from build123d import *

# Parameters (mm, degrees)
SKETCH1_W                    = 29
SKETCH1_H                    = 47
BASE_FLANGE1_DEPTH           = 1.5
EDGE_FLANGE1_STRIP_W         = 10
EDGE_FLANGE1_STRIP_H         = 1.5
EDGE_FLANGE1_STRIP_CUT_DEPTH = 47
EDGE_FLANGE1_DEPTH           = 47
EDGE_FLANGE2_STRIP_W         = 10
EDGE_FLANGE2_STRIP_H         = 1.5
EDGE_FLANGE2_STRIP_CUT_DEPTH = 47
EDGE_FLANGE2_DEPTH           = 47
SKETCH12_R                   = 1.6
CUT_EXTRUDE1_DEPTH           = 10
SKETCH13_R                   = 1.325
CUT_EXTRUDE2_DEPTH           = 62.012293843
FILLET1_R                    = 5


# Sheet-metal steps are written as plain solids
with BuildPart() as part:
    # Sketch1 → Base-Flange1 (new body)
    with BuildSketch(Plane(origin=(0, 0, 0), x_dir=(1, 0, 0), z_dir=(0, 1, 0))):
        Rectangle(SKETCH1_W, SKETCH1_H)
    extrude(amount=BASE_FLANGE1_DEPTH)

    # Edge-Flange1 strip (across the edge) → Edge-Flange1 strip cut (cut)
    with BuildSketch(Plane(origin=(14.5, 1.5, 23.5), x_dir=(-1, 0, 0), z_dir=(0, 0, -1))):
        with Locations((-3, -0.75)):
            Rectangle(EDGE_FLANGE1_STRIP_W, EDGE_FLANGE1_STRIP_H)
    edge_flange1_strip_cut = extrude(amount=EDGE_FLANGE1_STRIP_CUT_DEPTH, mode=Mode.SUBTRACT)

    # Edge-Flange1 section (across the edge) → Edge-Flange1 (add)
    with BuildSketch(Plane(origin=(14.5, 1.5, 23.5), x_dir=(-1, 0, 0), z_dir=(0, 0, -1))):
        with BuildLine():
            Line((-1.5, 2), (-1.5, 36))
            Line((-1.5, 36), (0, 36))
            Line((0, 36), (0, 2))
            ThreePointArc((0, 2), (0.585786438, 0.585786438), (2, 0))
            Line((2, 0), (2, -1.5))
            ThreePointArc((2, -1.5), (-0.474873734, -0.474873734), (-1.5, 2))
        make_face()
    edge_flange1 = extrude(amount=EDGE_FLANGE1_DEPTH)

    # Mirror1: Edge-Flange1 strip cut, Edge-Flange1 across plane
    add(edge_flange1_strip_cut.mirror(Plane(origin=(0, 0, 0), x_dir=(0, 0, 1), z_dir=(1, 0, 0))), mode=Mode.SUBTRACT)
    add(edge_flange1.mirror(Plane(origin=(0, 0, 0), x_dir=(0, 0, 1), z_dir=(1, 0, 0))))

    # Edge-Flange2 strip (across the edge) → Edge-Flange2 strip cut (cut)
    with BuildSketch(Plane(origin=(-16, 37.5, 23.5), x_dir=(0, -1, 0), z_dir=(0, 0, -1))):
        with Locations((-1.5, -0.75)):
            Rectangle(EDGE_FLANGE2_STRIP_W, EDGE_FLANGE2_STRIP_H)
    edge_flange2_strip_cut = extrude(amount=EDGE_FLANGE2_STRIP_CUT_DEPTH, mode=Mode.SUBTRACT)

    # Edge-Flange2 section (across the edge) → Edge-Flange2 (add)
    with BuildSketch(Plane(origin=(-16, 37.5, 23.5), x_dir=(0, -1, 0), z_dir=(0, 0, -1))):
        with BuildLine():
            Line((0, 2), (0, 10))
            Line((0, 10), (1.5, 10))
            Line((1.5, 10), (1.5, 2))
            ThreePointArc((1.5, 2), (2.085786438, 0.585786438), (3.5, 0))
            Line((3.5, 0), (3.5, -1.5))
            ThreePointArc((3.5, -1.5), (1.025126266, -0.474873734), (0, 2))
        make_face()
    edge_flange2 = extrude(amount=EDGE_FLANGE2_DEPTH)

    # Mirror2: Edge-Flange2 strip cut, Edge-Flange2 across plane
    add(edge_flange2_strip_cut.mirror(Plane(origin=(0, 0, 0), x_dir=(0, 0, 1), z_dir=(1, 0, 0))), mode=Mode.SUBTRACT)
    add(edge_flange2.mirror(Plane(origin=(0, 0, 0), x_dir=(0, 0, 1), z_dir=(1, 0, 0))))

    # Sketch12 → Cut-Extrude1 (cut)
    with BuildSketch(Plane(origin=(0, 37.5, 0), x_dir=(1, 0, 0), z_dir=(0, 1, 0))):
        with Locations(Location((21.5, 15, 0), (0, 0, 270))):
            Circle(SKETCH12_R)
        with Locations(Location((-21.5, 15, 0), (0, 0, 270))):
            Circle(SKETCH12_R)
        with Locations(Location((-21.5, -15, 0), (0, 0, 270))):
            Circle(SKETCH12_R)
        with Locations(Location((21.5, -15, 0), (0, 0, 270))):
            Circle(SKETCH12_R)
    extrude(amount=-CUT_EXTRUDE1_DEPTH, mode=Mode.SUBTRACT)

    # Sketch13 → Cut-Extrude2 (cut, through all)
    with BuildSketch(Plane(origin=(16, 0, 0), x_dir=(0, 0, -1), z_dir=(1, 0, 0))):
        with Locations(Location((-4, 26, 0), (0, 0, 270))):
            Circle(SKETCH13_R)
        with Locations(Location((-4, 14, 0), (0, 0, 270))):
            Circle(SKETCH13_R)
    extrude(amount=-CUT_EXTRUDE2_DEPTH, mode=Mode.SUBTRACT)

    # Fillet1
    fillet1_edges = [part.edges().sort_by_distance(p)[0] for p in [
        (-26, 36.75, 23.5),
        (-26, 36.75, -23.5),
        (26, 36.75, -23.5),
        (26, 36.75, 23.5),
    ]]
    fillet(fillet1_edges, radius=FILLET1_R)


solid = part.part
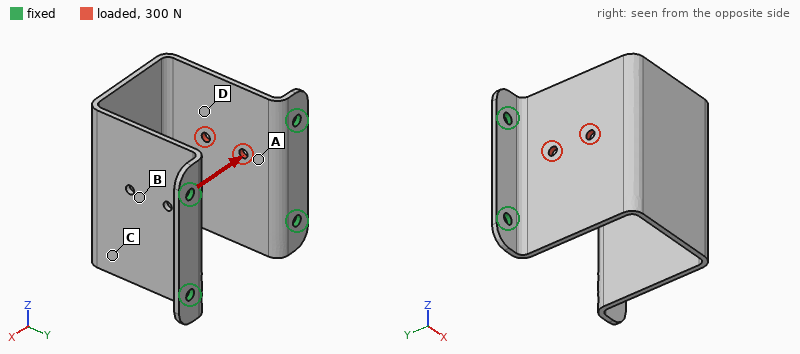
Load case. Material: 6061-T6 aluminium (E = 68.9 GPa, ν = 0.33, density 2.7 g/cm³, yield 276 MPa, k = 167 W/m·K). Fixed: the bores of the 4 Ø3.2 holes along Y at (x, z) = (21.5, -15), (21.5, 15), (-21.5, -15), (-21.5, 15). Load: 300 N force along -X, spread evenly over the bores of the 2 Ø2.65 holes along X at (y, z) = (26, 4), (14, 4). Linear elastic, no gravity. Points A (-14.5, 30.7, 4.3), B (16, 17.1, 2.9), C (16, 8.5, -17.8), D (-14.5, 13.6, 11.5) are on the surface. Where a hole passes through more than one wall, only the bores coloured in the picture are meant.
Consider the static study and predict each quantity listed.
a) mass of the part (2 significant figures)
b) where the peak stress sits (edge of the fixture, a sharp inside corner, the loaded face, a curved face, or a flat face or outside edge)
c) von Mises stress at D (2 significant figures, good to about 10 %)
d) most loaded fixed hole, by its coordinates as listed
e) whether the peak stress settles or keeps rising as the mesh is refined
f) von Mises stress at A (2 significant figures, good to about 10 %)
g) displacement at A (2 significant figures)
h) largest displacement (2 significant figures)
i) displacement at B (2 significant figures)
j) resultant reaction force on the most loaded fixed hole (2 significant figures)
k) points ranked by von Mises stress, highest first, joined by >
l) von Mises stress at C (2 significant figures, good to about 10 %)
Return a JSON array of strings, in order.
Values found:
["22 g", "edge of the fixture", "85 MPa", "(-21.5, 15)", "keeps rising", "59 MPa", "0.15 mm", "0.49 mm", "0.26 mm", "150 N", "D > A > C > B", "33 MPa"]
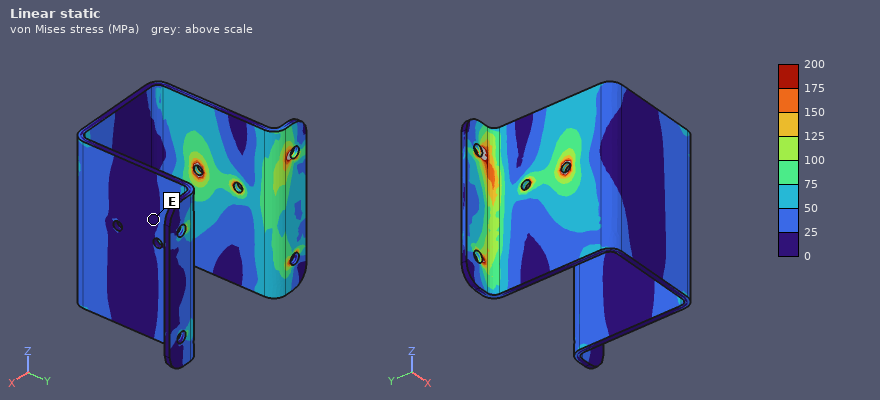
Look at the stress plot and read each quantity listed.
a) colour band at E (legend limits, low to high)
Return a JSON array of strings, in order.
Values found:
["0 to 25 MPa"]
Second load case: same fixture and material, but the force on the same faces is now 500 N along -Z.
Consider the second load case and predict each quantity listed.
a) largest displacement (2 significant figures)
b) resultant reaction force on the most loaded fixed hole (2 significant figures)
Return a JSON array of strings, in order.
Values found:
["0.14 mm", "370 N"]
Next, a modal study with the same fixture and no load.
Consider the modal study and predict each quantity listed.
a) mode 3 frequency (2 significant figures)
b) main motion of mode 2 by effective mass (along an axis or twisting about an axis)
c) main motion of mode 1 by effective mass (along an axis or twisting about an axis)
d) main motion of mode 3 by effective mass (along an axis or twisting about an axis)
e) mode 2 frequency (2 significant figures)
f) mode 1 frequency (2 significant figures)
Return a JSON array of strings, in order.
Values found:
["3000 Hz", "twisting about Y", "along X", "along Z", "2400 Hz", "870 Hz"]
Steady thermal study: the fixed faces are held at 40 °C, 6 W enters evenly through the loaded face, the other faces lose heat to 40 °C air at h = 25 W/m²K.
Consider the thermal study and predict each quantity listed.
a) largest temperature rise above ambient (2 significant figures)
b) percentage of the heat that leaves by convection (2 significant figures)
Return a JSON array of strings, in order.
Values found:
["12 K", "19 %"]
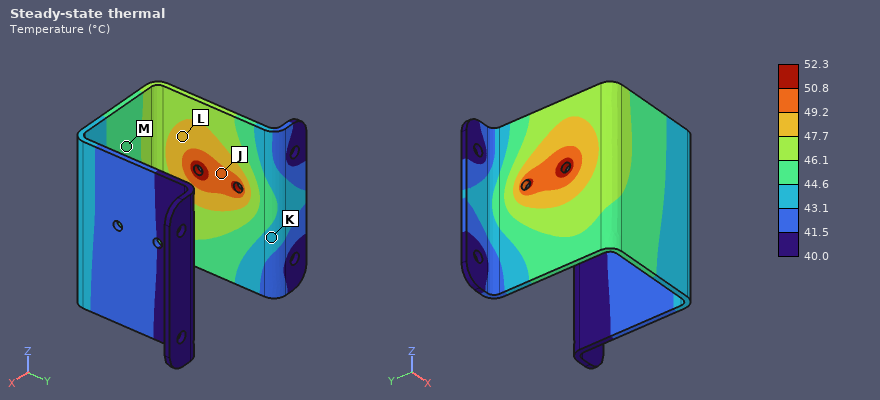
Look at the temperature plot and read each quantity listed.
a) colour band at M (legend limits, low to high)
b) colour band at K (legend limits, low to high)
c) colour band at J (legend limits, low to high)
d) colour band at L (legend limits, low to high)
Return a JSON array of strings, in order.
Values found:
["44.6 to 46.1 °C", "43.1 to 44.6 °C", "49.2 to 50.8 °C", "47.7 to 49.2 °C"]
